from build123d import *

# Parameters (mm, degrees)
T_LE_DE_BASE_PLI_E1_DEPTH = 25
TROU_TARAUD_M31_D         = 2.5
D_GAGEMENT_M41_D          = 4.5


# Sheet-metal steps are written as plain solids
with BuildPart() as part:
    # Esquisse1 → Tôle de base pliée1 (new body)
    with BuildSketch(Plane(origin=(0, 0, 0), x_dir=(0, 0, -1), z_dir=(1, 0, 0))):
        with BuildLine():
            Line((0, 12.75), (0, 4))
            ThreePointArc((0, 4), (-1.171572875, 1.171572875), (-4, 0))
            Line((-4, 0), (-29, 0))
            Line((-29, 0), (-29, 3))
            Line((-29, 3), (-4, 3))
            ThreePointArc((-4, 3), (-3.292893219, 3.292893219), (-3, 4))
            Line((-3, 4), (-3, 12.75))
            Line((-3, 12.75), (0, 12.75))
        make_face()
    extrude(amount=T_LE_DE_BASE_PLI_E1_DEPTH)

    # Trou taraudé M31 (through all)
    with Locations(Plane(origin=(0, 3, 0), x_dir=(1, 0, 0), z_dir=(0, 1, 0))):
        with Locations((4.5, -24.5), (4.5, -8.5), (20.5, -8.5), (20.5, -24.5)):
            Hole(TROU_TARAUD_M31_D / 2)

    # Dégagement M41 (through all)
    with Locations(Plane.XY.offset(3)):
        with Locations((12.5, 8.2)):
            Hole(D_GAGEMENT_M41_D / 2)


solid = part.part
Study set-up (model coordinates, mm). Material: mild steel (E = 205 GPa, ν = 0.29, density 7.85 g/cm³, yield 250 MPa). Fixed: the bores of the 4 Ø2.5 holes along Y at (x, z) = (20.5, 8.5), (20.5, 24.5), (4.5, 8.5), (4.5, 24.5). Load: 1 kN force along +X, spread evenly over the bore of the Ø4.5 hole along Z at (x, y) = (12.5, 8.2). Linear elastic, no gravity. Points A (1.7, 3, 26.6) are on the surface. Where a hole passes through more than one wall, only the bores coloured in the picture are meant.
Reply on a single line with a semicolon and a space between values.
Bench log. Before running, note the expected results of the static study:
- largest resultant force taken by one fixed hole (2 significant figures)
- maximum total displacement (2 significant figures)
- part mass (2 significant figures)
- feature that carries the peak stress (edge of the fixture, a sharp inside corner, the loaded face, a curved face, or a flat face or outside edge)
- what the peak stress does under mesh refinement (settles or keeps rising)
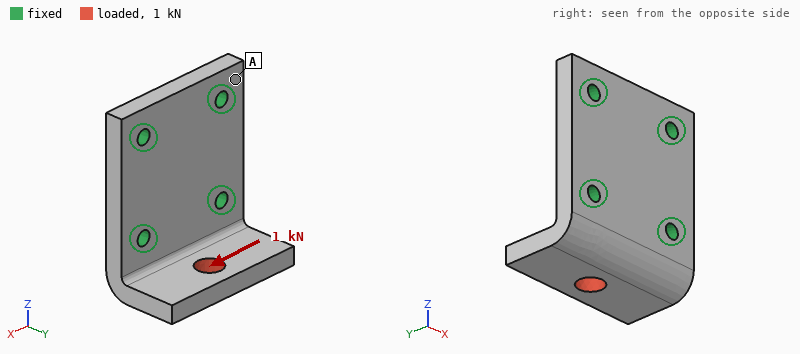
720 N; 15 µm; 21 g; edge of the fixture; keeps rising
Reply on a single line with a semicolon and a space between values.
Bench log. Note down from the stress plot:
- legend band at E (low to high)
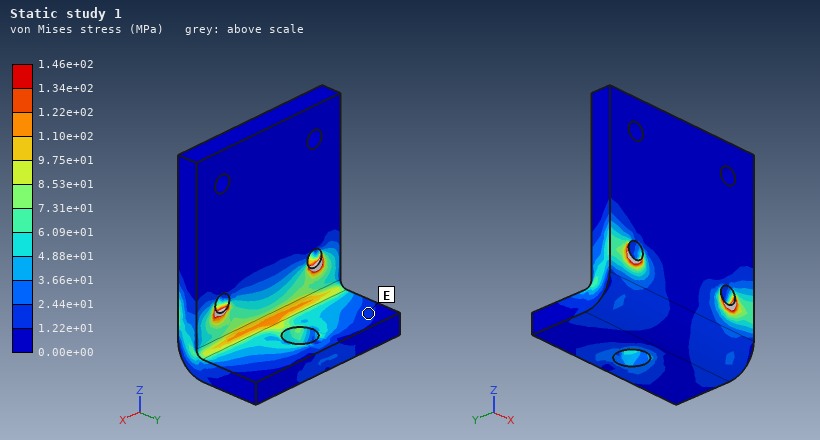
1.22e+01 to 2.44e+01 MPa
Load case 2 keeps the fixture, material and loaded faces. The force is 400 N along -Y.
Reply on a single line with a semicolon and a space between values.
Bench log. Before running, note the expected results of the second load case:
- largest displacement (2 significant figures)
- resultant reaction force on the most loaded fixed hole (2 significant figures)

13 µm; 220 N
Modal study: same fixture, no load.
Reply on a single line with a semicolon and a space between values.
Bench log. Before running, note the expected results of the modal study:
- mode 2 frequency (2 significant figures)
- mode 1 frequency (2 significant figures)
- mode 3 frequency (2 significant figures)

16 kHz; 10 kHz; 26 kHz
